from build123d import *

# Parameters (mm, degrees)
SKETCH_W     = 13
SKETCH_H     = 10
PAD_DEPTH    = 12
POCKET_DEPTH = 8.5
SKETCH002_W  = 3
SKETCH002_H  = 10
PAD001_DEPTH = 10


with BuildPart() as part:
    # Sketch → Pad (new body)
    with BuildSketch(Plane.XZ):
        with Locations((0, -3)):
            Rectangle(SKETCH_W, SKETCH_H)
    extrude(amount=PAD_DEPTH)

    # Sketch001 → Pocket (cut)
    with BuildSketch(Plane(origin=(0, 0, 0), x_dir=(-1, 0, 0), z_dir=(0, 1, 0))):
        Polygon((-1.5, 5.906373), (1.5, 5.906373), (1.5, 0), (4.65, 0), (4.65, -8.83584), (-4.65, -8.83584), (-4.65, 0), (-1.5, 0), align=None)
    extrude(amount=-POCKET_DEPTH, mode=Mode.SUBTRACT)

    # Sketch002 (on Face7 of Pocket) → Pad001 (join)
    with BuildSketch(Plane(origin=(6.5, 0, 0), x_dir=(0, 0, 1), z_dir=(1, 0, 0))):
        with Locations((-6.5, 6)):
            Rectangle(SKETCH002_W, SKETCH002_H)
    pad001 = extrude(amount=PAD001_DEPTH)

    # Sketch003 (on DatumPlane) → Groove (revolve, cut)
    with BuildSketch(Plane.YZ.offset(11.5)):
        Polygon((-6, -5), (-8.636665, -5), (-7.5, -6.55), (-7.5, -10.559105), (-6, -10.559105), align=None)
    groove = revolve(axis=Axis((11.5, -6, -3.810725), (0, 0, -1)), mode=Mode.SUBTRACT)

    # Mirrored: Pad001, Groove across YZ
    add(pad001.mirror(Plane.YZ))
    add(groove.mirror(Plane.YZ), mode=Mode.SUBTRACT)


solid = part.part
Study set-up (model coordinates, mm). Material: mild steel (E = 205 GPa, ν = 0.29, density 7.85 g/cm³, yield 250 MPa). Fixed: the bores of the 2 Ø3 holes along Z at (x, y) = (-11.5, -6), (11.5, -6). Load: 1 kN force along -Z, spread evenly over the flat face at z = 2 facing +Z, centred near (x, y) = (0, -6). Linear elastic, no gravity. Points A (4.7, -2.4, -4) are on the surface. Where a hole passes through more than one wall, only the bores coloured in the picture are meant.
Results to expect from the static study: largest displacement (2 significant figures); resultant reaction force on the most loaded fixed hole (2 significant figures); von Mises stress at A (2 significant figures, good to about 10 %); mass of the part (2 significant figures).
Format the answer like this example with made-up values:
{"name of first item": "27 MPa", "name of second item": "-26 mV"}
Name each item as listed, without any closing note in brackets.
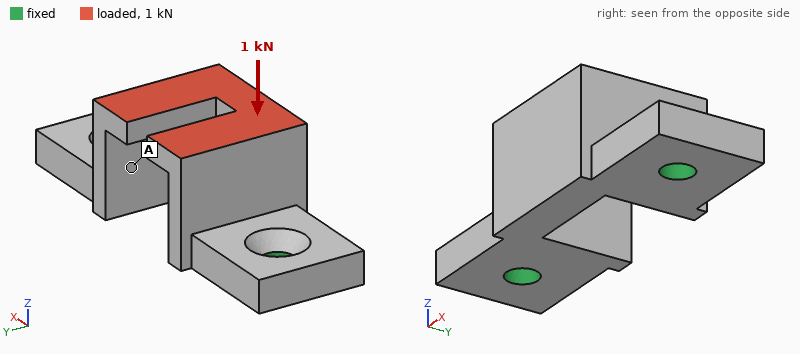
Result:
{"largest displacement": "14 µm", "resultant reaction force on the most loaded fixed hole": "570 N", "von Mises stress at A": "33 MPa", "mass of the part": "11 g"}
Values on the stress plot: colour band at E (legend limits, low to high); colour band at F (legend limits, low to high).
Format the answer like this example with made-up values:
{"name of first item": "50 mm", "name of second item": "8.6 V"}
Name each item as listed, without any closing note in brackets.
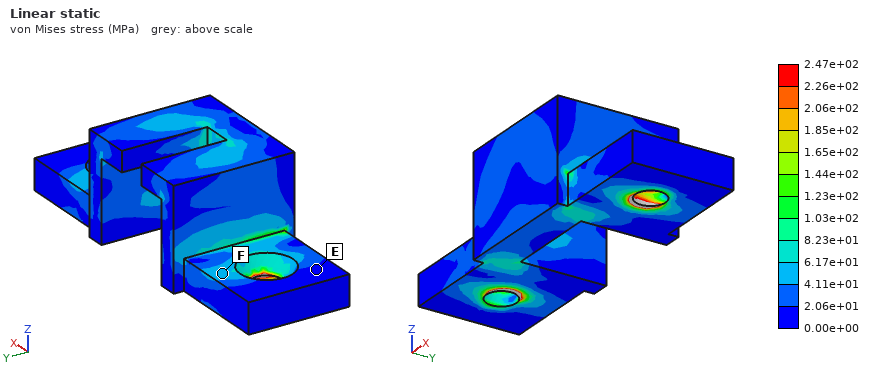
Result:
{"colour band at E": "0.00e+00 to 2.06e+01 MPa", "colour band at F": "4.11e+01 to 6.17e+01 MPa"}
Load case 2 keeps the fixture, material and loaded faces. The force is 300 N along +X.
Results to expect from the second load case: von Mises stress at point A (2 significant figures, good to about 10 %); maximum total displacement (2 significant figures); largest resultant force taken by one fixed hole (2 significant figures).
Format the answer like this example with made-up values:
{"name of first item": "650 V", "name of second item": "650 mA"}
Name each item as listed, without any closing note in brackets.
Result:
{"von Mises stress at point A": "32 MPa", "maximum total displacement": "9.9 µm", "largest resultant force taken by one fixed hole": "200 N"}
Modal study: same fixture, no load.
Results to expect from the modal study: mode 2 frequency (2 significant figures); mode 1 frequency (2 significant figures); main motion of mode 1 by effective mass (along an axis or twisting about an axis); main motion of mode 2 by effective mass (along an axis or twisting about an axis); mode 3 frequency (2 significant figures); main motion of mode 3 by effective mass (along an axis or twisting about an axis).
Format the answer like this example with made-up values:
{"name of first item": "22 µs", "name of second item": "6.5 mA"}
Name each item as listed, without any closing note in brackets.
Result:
{"mode 2 frequency": "20 kHz", "mode 1 frequency": "11 kHz", "main motion of mode 1 by effective mass": "along Y", "main motion of mode 2 by effective mass": "along X", "mode 3 frequency": "21 kHz", "main motion of mode 3 by effective mass": "along Z"}
